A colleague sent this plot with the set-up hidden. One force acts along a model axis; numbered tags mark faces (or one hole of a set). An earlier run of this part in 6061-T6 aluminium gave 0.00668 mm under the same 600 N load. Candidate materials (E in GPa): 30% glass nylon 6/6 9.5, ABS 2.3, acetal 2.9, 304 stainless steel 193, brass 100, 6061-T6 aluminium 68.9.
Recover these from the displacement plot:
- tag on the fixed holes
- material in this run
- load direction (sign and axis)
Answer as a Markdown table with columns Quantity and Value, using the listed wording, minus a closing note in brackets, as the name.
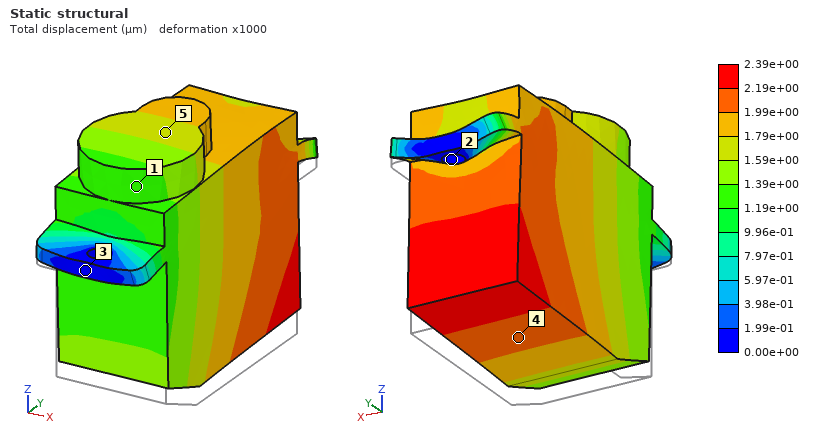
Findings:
| Quantity | Value |
|---|---|
| tag on the fixed holes | 2 |
| material in this run | 304 stainless steel |
| load direction | +Z |
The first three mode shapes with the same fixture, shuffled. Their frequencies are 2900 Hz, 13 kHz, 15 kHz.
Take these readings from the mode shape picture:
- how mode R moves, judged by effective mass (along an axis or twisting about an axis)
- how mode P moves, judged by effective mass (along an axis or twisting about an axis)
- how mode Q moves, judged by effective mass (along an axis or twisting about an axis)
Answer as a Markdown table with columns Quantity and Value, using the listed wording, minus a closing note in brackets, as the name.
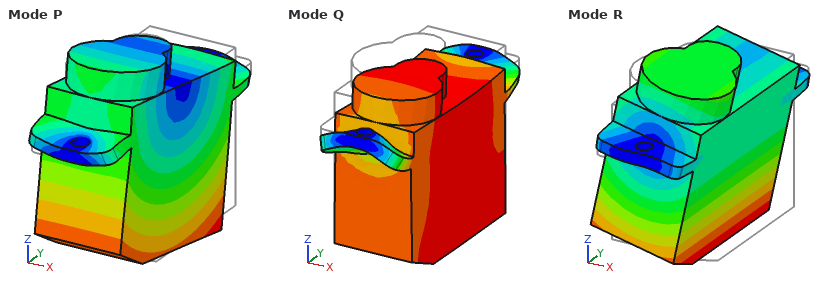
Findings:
| Quantity | Value |
|---|---|
| how mode R moves, judged by effective mass | along X |
| how mode P moves, judged by effective mass | along Y |
| how mode Q moves, judged by effective mass | along Z |
